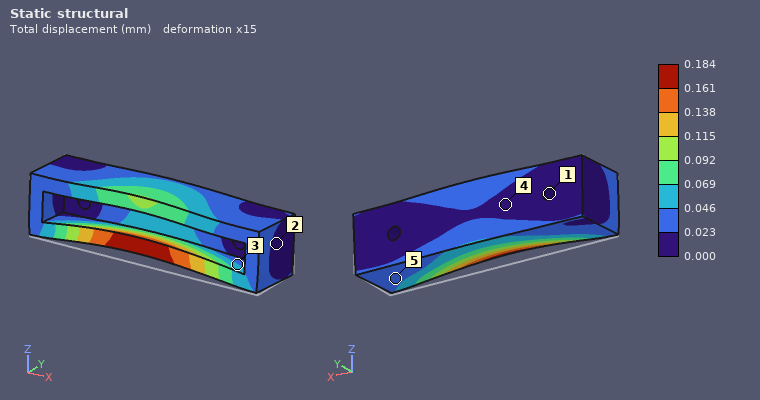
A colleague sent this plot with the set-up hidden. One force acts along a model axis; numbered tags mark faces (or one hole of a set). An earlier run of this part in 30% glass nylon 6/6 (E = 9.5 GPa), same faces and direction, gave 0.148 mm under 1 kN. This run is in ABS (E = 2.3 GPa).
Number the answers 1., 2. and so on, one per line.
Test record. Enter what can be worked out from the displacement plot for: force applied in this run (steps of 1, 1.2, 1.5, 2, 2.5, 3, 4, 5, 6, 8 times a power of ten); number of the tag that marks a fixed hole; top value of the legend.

1. 300 N
2. 1
3. 0.184 mm
